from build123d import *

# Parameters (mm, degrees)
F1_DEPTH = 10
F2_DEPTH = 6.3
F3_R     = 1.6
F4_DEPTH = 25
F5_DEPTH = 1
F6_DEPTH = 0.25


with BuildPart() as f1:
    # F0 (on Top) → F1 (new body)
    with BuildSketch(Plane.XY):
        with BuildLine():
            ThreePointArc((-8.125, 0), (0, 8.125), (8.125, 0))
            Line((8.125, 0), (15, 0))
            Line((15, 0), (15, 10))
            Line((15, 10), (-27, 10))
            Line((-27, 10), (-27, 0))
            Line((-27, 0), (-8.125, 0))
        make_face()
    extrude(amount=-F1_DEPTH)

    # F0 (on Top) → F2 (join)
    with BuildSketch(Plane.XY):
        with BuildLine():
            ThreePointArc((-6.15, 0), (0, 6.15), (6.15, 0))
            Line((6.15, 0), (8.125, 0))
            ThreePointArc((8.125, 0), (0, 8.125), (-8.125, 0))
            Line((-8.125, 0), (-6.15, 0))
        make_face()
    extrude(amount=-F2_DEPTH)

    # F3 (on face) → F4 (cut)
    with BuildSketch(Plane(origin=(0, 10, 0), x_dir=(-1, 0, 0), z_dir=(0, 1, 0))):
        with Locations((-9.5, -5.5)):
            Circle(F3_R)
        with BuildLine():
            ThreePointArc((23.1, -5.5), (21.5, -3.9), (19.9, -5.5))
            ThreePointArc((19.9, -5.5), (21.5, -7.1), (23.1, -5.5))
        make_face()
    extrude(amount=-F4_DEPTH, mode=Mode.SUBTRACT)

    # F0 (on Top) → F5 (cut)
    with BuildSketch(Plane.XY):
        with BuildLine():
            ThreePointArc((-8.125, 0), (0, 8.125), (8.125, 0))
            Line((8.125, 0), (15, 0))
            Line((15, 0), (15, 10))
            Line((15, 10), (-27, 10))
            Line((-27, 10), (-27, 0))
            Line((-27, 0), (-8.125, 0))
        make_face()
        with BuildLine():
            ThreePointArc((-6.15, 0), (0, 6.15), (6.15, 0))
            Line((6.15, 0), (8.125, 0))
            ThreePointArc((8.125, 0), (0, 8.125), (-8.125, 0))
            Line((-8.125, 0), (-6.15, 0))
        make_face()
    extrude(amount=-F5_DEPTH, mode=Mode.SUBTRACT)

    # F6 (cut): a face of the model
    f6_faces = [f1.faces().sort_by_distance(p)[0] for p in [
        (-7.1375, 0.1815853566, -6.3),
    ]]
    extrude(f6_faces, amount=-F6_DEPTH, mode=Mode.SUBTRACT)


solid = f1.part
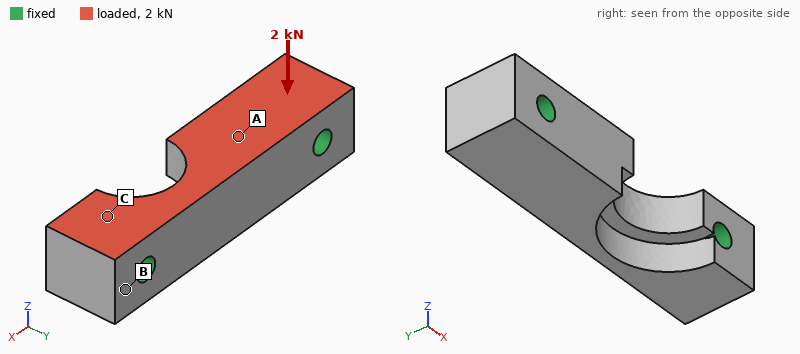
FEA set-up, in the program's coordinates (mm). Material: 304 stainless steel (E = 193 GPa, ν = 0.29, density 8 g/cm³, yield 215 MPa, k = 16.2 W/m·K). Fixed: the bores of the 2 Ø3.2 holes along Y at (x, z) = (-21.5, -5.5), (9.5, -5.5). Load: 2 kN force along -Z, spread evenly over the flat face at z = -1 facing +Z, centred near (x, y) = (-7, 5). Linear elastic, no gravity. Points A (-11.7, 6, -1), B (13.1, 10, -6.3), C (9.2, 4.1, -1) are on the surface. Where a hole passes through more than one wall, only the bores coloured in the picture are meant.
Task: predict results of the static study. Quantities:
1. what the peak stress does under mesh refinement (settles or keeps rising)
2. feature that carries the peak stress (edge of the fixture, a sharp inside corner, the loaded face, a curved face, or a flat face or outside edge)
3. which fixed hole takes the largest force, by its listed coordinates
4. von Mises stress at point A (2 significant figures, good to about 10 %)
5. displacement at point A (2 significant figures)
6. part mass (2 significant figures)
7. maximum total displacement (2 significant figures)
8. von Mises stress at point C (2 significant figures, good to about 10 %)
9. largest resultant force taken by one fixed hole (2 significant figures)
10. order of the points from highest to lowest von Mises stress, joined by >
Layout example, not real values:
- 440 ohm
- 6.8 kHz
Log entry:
- keeps rising
- edge of the fixture
- (-21.5, -5.5)
- 12 MPa
- 2.6 µm
- 23 g
- 4.1 µm
- 19 MPa
- 1.1 kN
- C > A > B
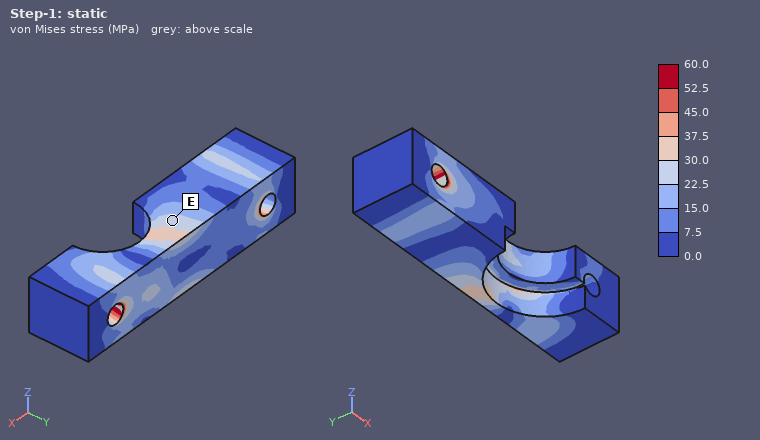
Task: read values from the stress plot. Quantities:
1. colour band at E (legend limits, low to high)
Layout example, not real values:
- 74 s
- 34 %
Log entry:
- 22.5 to 30.0 MPa
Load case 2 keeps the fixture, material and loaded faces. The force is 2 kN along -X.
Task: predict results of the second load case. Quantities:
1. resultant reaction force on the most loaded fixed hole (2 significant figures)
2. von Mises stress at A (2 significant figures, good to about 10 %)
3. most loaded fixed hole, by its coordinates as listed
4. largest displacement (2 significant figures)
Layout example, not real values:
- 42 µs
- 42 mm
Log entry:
- 1.2 kN
- 12 MPa
- (-21.5, -5.5)
- 2.0 µm
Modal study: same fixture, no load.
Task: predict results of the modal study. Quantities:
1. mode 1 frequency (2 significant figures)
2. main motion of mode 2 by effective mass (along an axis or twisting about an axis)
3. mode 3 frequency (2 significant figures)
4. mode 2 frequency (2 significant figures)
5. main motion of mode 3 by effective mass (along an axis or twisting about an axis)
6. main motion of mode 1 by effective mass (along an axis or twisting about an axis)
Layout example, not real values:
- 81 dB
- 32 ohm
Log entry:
- 28 kHz
- along Y
- 45 kHz
- 31 kHz
- twisting about X
- along Z
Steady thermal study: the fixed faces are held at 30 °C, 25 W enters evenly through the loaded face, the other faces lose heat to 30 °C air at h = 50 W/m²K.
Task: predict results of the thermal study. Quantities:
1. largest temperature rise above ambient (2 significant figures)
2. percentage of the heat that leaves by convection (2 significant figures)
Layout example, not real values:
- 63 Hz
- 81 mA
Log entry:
- 65 K
- 6.0 %
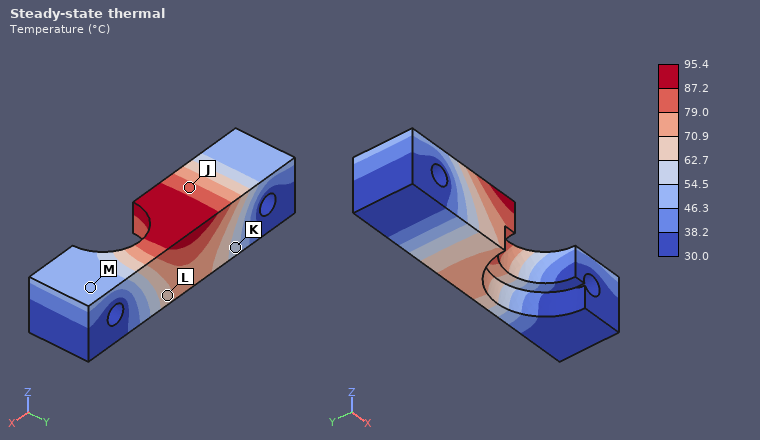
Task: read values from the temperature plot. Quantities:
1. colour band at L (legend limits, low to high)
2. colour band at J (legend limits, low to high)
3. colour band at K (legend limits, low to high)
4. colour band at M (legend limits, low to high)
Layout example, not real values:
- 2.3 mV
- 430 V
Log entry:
- 62.7 to 70.9 °C
- 79.0 to 87.2 °C
- 54.5 to 62.7 °C
- 46.3 to 54.5 °C
